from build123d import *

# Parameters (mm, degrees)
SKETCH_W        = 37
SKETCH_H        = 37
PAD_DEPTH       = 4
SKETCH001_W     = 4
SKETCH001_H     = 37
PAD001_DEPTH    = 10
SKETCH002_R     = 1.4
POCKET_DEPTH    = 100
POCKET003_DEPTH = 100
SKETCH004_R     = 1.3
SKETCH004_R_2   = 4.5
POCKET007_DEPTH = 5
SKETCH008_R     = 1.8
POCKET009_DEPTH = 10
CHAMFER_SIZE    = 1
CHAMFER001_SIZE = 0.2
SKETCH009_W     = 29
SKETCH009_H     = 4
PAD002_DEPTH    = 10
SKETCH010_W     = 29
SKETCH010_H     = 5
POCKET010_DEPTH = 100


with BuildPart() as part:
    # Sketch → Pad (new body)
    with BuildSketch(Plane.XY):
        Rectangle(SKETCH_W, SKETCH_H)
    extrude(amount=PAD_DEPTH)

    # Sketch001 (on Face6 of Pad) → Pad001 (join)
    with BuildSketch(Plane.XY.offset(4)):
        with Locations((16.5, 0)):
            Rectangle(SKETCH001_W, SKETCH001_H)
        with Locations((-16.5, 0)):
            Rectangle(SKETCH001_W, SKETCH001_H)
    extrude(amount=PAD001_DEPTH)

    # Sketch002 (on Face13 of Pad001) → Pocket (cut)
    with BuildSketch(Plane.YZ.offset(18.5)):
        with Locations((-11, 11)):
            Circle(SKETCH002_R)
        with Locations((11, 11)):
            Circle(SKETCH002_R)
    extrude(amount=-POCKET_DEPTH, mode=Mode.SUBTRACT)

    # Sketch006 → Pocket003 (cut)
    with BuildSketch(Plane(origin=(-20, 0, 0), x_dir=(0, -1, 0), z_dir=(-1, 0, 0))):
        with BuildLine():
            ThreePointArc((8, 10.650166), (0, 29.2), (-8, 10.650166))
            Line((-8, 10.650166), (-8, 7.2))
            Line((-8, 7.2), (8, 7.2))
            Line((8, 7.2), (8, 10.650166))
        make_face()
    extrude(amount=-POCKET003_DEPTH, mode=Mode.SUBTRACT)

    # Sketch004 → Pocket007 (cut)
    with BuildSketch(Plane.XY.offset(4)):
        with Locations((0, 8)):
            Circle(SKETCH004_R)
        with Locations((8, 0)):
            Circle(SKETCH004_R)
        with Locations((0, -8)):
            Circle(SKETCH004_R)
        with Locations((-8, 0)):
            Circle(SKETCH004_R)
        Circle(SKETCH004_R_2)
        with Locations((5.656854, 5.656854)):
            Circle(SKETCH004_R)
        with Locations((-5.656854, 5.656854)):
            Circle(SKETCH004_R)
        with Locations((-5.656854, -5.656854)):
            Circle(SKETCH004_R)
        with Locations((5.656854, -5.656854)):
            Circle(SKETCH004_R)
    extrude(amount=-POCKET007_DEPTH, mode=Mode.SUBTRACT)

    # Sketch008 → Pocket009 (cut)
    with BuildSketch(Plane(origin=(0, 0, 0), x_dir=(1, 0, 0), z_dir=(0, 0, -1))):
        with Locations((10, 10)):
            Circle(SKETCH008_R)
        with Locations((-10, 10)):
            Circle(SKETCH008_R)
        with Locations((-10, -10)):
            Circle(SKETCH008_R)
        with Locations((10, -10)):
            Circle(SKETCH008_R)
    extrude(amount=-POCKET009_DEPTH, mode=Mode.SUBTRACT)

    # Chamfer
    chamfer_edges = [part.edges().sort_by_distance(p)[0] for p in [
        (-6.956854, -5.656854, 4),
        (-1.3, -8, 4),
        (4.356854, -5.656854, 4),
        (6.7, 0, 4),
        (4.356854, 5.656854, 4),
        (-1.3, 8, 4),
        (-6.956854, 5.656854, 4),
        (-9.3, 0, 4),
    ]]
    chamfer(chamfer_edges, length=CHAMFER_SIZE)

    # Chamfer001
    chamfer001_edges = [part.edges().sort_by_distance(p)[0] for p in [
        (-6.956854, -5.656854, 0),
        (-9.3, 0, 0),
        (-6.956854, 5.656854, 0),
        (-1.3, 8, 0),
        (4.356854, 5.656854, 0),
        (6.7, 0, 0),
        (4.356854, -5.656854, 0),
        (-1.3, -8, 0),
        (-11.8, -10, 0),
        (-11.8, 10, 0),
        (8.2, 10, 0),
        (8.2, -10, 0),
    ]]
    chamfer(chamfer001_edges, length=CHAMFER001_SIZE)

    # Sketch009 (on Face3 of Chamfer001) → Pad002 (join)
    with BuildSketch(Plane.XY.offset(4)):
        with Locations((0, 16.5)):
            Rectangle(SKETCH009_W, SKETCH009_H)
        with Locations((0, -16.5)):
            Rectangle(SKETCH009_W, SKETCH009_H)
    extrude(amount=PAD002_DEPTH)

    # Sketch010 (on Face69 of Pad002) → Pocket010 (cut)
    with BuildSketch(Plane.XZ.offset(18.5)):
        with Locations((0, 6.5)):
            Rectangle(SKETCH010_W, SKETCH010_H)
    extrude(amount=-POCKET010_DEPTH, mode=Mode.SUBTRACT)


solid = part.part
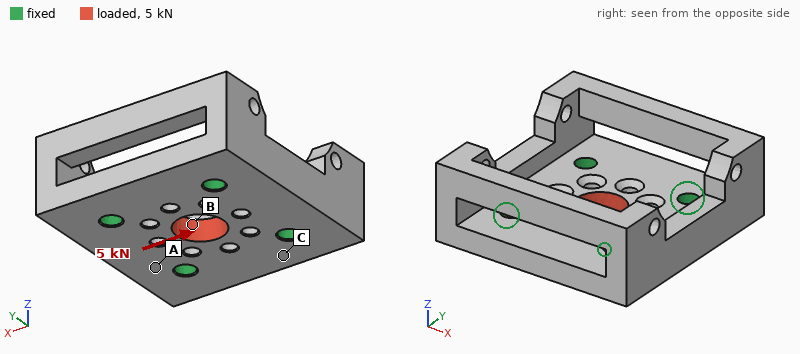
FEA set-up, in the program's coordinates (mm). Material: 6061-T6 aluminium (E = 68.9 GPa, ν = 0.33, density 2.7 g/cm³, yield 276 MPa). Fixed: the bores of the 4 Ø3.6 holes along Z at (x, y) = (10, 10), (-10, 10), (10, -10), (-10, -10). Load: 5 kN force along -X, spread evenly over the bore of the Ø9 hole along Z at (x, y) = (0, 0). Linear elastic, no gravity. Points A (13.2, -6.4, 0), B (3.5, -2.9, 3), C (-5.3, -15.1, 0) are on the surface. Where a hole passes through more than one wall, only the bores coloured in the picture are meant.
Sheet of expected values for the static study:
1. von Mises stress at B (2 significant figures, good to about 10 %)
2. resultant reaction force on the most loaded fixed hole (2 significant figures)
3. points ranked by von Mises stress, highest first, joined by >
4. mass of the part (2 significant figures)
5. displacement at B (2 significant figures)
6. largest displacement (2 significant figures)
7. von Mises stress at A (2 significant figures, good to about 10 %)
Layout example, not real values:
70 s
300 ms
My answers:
64 MPa
1.3 kN
B > A > C
21 g
9.3 µm
10 µm
29 MPa
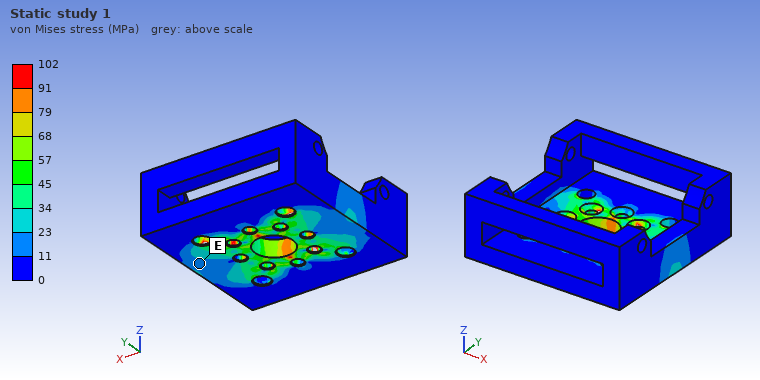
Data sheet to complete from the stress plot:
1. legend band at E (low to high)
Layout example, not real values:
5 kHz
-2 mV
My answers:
11 to 23 MPa
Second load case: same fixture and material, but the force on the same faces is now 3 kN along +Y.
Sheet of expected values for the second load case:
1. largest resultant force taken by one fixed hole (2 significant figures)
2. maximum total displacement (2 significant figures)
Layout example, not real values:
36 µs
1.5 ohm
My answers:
780 N
6.3 µm
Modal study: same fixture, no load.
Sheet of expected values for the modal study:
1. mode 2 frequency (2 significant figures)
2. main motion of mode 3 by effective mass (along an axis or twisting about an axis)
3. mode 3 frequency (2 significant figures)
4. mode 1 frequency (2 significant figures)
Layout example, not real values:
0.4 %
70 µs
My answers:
12 kHz
along X
13 kHz
12 kHz
